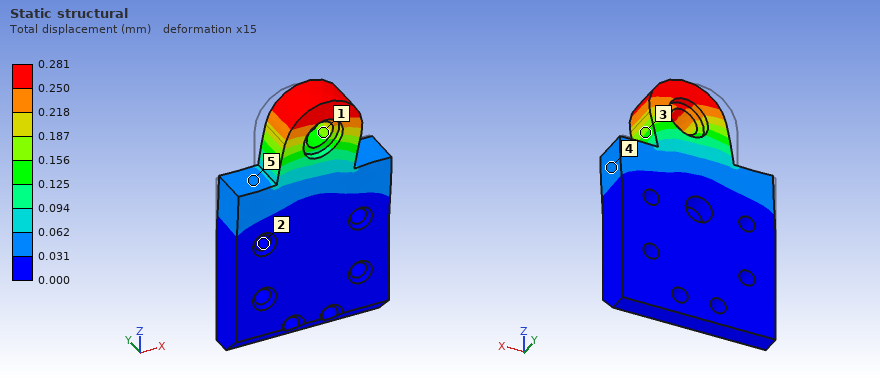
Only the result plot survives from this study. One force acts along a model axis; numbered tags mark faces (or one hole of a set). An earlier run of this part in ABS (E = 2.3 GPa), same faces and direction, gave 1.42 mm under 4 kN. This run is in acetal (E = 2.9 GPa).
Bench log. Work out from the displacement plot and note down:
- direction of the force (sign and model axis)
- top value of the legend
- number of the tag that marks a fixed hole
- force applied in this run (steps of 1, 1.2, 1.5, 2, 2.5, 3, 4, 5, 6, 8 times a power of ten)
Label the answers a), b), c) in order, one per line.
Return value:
a) +X
b) 0.281 mm
c) 2
d) 1 kN
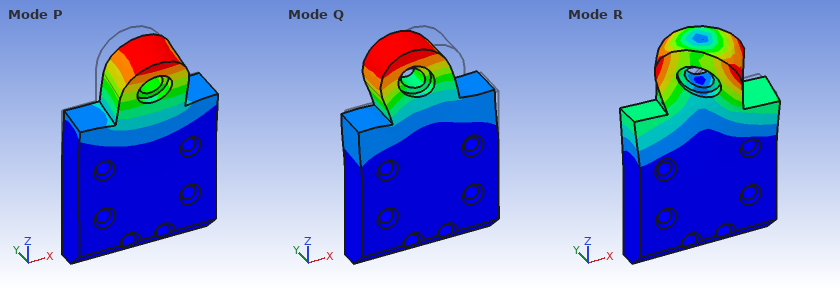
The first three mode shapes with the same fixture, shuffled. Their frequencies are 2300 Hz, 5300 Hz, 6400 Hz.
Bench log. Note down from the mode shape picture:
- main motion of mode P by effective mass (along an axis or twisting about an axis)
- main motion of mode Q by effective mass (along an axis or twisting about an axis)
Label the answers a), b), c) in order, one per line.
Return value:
a) along Y
b) along X
